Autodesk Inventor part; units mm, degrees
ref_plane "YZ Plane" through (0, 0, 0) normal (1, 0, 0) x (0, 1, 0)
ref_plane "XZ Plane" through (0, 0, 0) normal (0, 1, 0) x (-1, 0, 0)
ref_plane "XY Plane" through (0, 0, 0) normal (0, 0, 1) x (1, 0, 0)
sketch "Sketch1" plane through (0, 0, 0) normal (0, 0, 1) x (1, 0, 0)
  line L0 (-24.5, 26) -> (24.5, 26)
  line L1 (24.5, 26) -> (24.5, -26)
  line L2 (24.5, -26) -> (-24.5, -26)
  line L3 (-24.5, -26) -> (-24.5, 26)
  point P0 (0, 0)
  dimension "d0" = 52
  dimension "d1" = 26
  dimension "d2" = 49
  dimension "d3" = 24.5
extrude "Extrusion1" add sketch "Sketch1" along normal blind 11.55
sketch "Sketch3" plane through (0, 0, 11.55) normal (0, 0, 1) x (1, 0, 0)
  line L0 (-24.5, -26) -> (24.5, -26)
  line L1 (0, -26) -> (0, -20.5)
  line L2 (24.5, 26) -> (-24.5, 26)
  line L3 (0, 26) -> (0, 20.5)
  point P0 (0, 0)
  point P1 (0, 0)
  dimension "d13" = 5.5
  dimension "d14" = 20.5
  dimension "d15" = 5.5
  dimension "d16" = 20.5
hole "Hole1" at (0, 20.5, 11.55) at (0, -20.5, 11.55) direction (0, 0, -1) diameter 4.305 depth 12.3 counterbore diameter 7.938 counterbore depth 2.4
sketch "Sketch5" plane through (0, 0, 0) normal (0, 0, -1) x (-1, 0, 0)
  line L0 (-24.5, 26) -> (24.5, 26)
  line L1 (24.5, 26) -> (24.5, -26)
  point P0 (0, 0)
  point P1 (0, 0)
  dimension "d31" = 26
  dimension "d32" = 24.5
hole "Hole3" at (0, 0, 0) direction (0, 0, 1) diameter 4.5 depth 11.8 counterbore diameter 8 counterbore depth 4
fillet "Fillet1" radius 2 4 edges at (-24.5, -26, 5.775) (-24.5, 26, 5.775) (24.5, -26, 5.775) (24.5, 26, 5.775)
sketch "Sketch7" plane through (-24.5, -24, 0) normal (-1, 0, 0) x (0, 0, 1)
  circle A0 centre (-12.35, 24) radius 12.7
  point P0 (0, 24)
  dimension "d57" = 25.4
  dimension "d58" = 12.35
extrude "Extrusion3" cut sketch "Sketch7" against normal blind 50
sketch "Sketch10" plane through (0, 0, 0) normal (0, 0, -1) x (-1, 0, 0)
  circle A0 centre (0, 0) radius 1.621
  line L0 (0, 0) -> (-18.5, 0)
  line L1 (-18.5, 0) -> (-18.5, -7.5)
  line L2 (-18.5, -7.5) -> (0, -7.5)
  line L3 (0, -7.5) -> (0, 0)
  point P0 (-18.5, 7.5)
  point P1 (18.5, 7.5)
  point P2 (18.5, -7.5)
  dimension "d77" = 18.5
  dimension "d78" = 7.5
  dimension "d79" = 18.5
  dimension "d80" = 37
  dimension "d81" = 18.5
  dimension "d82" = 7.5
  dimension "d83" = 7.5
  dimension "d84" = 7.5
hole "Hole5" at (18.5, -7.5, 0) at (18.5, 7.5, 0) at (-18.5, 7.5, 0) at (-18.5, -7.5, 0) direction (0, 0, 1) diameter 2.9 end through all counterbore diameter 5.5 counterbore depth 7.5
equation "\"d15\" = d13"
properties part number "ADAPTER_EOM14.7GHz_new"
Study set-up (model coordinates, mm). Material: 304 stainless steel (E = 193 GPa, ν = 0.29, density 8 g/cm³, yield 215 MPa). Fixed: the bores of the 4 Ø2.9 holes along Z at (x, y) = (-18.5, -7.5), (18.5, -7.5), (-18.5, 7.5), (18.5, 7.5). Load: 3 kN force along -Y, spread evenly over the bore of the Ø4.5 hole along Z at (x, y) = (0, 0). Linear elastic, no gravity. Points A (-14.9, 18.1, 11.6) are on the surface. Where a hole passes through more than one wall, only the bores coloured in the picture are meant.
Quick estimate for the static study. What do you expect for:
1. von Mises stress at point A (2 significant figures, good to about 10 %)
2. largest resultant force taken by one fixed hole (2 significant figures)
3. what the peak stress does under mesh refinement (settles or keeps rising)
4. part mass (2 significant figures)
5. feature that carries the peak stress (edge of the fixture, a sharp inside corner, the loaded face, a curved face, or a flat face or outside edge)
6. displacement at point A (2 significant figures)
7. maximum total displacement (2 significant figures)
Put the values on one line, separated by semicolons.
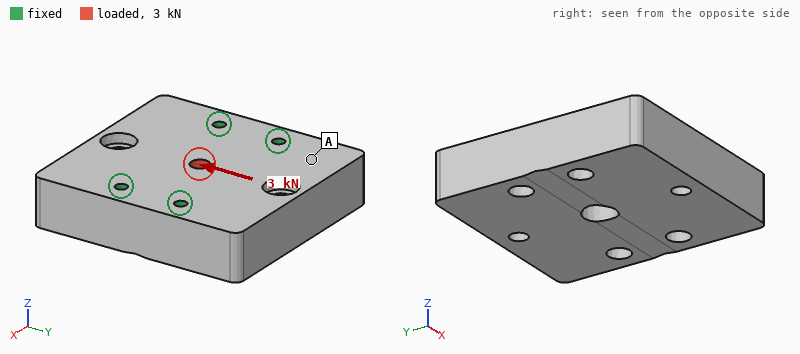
4.6 MPa; 770 N; keeps rising; 220 g; edge of the fixture; 0.63 µm; 1.9 µm
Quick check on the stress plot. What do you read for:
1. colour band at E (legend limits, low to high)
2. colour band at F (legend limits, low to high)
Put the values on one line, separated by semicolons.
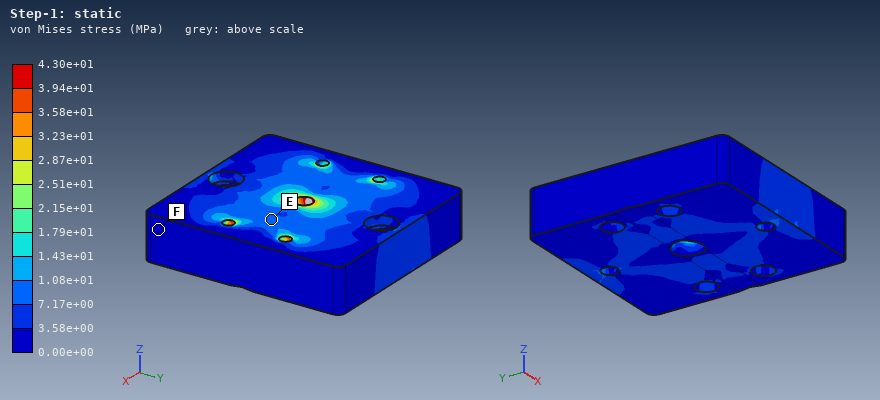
7.17e+00 to 1.08e+01 MPa; 0.00e+00 to 3.58e+00 MPa
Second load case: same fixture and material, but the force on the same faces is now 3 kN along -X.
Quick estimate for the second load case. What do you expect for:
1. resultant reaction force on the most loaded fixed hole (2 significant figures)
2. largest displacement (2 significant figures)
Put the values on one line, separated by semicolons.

760 N; 1.5 µm
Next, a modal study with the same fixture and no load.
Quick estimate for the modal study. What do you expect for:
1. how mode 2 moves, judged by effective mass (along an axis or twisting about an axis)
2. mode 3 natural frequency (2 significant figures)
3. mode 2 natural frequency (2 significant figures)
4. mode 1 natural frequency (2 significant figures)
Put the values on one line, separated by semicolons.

along Z; 17 kHz; 12 kHz; 9100 Hz
